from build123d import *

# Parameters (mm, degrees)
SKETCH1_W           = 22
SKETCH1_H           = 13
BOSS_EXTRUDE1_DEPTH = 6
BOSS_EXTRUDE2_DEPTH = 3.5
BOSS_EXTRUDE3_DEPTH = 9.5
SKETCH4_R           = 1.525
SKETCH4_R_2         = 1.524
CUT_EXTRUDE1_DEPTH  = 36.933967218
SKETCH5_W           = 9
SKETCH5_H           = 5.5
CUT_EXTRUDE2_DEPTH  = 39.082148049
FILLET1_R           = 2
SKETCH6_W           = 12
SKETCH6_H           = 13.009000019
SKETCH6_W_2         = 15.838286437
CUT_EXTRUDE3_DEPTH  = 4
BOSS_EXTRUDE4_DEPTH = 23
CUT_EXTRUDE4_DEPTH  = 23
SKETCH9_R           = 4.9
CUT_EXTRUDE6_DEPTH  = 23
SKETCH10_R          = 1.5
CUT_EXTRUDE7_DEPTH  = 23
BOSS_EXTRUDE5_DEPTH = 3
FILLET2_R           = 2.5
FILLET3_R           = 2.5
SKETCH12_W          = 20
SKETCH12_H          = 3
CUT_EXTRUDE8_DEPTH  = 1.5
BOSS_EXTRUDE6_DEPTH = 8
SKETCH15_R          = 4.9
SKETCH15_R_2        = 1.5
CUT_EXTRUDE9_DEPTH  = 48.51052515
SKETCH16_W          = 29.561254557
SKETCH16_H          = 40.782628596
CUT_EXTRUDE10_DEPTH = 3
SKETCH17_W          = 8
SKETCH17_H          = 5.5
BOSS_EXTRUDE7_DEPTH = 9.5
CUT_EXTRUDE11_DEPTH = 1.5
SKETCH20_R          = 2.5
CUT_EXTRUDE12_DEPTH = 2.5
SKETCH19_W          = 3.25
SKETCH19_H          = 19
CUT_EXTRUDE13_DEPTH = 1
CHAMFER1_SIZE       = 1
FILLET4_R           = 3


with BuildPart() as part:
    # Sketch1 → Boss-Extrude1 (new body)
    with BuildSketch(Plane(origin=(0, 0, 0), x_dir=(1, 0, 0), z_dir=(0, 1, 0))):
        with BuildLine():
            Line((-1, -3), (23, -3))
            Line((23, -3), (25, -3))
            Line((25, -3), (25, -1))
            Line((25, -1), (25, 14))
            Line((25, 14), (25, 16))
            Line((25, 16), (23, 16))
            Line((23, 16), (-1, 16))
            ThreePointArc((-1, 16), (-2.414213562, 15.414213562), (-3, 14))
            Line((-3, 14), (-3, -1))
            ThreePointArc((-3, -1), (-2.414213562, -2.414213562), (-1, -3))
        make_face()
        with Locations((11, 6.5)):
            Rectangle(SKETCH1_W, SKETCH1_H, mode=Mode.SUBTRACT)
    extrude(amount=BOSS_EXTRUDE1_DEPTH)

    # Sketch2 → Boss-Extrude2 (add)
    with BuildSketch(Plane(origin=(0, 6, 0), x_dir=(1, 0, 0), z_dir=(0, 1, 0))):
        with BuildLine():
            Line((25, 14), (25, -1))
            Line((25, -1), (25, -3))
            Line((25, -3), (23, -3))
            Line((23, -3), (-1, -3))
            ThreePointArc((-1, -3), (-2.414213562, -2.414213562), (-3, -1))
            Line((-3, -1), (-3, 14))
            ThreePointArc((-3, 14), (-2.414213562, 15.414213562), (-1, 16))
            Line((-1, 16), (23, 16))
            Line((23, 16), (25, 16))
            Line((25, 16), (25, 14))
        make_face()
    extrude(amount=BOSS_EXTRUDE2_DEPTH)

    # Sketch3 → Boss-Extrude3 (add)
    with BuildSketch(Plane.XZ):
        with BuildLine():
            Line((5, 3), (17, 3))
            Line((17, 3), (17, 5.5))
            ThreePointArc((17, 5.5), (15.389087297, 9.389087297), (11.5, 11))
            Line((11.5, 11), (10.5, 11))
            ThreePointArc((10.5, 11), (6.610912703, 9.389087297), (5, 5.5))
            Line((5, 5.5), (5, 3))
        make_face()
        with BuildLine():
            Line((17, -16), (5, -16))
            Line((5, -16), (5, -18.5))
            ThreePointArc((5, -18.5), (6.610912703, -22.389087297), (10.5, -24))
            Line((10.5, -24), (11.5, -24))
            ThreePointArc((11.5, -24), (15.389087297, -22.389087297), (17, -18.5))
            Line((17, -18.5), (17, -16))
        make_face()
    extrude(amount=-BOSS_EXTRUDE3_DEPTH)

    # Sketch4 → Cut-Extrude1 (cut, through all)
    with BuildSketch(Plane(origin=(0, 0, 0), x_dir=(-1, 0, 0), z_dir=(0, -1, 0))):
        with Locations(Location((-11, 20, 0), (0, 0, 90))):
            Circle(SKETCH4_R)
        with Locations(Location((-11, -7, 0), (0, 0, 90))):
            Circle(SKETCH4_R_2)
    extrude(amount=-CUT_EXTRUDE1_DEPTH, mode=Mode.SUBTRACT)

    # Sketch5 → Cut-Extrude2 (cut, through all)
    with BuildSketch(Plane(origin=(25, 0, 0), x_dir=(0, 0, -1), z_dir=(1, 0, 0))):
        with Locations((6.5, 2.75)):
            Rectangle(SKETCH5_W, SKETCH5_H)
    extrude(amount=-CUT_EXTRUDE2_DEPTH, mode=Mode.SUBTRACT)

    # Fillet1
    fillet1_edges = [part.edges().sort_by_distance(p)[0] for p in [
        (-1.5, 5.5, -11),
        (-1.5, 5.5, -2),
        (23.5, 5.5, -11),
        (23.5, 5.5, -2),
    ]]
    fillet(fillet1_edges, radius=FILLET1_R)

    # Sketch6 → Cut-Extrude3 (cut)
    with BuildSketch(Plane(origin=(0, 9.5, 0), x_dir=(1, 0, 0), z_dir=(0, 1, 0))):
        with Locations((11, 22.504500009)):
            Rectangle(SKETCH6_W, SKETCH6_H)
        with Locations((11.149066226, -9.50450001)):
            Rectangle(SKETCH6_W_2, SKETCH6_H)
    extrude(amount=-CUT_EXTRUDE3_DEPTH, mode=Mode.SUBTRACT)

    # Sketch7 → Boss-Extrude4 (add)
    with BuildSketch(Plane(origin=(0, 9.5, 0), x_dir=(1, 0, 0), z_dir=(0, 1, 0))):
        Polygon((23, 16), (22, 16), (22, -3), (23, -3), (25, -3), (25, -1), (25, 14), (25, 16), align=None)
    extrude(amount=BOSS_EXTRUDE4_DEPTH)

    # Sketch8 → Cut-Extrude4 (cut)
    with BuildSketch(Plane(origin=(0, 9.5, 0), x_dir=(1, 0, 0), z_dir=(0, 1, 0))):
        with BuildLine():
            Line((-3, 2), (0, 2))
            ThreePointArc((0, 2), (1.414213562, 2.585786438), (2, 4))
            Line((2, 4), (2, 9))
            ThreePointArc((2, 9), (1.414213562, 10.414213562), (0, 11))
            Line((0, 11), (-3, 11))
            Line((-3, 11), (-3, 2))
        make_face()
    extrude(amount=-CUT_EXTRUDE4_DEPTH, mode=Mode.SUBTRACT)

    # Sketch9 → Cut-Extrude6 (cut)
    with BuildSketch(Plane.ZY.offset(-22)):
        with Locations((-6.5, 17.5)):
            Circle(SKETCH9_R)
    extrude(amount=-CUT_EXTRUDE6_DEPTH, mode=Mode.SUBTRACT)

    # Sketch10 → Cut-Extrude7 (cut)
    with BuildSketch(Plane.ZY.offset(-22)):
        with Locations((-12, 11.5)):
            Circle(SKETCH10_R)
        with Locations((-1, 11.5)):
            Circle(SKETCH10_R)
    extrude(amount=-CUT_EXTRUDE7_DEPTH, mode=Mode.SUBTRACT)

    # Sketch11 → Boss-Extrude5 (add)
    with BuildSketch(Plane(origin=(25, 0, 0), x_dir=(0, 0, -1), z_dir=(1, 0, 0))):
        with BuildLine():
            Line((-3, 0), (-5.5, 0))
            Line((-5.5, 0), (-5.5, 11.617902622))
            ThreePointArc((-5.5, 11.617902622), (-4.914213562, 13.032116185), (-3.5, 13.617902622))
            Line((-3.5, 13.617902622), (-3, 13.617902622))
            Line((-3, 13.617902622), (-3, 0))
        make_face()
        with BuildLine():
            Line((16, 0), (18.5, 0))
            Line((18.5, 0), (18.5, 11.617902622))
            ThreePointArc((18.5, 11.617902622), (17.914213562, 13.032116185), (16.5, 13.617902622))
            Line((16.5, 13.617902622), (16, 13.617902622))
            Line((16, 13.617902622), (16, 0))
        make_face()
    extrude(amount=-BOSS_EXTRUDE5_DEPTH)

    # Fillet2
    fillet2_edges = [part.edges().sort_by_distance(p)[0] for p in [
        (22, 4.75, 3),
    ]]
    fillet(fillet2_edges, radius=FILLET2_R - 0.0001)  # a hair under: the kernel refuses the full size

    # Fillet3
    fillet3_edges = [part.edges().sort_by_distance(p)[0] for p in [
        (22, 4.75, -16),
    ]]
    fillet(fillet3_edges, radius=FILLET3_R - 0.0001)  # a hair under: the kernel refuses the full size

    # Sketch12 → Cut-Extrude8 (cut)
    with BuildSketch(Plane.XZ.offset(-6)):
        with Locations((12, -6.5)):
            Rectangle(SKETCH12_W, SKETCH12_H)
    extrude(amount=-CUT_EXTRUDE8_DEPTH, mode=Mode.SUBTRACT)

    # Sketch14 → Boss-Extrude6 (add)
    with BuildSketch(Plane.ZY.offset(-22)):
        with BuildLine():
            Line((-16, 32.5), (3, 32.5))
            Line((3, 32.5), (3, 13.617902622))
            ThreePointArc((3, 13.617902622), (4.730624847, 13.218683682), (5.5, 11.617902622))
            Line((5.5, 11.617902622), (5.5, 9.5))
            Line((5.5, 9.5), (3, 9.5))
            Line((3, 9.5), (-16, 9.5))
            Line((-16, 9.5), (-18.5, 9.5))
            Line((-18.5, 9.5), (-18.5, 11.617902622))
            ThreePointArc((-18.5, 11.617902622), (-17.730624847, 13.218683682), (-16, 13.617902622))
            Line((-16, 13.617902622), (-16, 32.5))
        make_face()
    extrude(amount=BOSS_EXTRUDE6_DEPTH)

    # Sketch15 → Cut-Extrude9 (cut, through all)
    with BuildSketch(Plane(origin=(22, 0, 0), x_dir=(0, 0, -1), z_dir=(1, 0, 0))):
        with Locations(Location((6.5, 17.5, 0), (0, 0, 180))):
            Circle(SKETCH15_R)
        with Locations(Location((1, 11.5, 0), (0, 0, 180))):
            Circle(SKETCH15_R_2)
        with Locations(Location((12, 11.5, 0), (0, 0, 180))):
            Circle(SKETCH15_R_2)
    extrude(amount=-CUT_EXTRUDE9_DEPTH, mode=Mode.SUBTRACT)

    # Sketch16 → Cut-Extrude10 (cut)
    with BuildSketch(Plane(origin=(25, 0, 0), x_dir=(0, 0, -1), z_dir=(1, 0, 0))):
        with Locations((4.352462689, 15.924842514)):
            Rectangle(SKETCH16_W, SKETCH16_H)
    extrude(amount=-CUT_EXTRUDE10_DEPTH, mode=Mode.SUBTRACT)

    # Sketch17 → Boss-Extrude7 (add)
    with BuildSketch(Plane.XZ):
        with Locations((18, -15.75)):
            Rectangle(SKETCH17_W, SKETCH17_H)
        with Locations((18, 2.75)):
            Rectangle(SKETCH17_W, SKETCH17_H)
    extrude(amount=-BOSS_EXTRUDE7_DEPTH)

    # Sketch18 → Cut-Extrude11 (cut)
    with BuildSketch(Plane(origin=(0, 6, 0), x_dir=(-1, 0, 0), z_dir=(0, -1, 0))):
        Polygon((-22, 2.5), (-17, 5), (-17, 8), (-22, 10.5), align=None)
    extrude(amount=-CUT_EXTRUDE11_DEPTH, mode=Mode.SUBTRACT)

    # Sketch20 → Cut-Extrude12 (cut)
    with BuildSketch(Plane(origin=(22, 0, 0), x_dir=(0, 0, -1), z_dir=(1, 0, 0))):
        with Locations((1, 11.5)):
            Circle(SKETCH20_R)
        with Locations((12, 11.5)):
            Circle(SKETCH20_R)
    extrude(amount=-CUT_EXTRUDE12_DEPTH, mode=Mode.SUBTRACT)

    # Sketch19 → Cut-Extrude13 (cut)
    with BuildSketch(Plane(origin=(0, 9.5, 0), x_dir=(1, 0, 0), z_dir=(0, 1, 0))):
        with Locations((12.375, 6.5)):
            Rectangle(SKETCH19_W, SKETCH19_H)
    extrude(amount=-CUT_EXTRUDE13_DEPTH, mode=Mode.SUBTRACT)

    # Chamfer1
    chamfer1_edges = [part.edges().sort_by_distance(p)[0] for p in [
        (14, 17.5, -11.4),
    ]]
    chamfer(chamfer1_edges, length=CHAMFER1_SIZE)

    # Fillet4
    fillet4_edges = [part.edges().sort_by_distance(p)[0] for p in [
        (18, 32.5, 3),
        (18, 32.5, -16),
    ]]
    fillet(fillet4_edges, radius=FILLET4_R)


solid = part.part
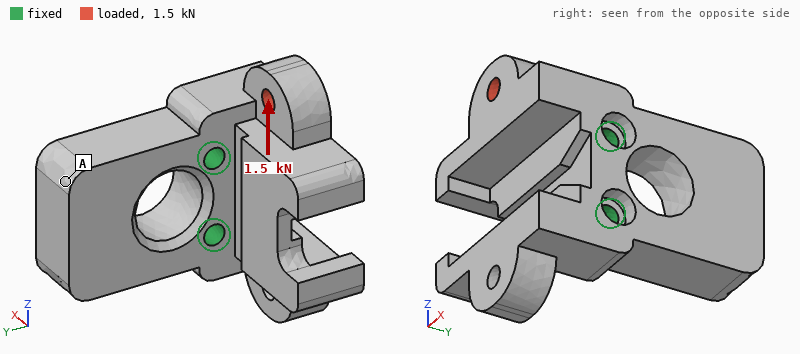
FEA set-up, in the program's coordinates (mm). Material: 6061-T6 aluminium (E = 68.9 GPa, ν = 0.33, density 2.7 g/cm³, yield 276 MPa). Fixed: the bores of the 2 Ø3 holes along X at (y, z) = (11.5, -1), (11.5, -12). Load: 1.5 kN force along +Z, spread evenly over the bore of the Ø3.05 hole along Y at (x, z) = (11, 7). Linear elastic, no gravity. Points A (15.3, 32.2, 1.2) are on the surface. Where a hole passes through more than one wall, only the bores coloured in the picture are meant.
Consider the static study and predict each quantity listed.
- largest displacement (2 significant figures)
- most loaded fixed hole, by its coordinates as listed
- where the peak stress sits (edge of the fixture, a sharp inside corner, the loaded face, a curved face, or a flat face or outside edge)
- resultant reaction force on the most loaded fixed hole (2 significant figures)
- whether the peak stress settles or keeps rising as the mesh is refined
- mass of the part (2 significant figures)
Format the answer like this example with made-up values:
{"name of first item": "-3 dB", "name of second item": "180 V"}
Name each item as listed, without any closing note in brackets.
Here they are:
{"largest displacement": "84 µm", "most loaded fixed hole, by its coordinates as listed": "(11.5, -12)", "where the peak stress sits": "edge of the fixture", "resultant reaction force on the most loaded fixed hole": "1.2 kN", "whether the peak stress settles or keeps rising as the mesh is refined": "keeps rising", "mass of the part": "17 g"}
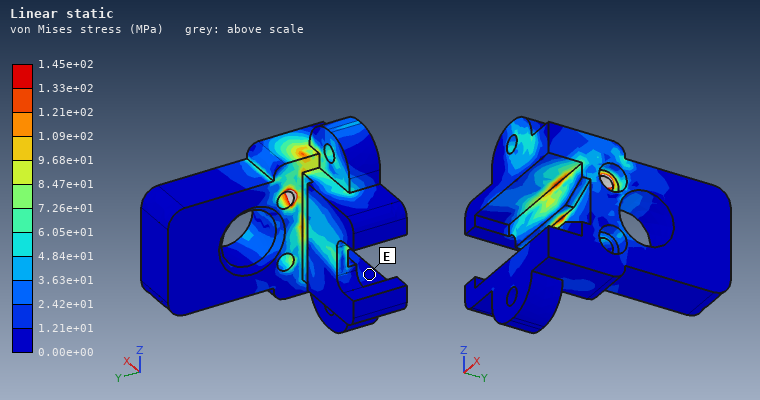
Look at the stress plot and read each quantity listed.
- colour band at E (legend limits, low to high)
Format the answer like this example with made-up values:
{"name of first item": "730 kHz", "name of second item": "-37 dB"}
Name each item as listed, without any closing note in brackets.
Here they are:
{"colour band at E": "0.00e+00 to 1.21e+01 MPa"}
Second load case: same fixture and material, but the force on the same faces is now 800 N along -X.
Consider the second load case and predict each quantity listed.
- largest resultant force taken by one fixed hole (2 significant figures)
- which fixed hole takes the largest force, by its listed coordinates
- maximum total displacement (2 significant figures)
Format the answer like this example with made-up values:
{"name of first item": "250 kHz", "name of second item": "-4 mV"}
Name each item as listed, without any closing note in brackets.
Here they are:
{"largest resultant force taken by one fixed hole": "1.1 kN", "which fixed hole takes the largest force, by its listed coordinates": "(11.5, -1)", "maximum total displacement": "51 µm"}
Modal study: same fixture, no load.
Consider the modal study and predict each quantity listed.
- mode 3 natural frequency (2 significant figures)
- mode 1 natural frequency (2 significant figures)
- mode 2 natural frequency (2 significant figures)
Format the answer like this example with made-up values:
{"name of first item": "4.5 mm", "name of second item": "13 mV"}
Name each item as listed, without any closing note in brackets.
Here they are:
{"mode 3 natural frequency": "11 kHz", "mode 1 natural frequency": "8100 Hz", "mode 2 natural frequency": "9900 Hz"}
